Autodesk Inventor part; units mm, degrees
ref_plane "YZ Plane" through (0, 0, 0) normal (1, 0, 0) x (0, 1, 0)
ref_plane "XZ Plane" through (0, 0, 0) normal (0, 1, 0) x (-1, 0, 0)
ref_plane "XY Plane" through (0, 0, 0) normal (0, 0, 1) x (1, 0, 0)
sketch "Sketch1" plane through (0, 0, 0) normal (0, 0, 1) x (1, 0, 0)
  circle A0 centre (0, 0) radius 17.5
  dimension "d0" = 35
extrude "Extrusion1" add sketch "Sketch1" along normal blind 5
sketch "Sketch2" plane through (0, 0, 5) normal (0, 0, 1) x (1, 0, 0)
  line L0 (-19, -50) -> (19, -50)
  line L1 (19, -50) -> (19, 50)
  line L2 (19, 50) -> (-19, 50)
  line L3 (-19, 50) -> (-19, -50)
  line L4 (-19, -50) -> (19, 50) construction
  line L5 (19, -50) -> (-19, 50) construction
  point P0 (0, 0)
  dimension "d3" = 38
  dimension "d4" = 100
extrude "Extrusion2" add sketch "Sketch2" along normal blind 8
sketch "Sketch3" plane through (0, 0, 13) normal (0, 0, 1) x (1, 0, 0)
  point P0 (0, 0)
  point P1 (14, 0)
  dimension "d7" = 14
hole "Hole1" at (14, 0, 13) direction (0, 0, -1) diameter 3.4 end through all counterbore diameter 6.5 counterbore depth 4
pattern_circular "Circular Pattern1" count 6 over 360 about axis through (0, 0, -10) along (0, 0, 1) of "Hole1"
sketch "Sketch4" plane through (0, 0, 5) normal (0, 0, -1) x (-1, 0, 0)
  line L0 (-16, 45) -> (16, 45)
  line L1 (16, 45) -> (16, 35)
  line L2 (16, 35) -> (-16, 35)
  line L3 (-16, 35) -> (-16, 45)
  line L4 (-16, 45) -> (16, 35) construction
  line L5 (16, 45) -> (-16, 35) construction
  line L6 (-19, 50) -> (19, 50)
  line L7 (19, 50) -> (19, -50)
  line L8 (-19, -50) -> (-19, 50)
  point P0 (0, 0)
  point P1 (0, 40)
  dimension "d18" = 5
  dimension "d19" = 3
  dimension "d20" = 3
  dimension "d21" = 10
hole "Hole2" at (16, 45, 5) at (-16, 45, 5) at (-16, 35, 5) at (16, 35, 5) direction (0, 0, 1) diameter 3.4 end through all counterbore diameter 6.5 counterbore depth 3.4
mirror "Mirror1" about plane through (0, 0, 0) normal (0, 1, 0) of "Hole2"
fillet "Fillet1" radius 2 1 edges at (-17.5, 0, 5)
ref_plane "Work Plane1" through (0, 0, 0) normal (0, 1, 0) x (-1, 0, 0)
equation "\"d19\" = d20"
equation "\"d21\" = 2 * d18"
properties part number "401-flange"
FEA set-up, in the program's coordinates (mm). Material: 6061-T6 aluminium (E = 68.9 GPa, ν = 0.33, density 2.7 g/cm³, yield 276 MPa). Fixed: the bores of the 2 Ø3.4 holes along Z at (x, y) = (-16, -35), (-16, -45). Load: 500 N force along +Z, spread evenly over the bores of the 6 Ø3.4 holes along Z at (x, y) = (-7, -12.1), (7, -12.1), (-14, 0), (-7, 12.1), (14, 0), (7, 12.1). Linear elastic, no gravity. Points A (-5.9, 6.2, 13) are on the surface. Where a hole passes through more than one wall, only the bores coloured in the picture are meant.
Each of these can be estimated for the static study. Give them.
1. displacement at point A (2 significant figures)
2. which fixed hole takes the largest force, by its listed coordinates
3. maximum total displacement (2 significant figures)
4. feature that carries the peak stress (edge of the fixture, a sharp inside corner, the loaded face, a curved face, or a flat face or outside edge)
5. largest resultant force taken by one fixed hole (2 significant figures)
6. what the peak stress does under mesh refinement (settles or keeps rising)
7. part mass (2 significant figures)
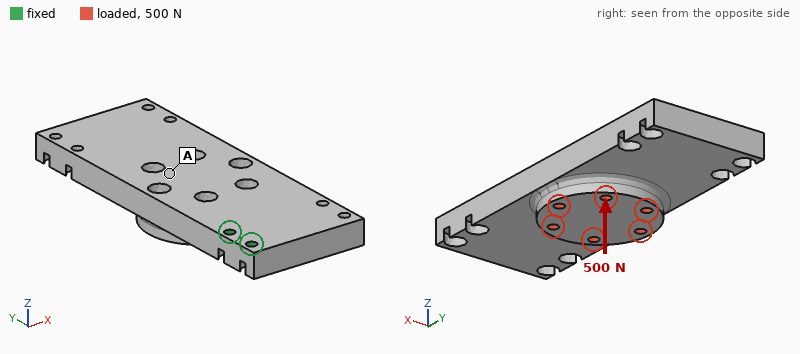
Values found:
0.23 mm
(-16, -35)
0.56 mm
edge of the fixture
1.5 kN
keeps rising
89 g
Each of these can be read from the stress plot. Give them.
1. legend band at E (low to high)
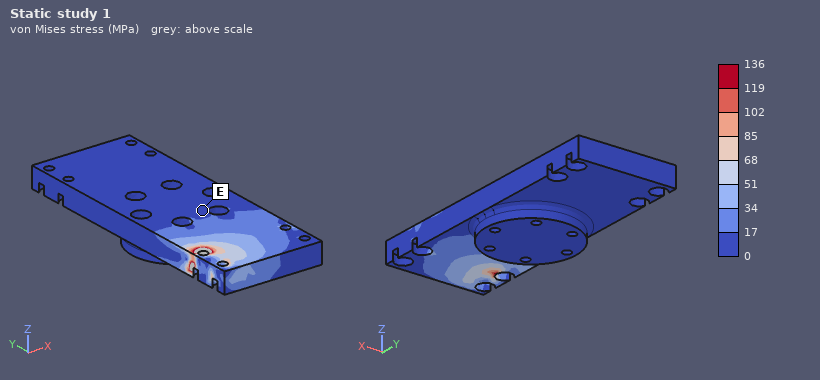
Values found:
0 to 17 MPa
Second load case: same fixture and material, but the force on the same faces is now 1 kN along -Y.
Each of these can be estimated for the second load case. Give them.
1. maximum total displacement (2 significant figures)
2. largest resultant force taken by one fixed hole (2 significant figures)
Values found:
0.15 mm
1.4 kN
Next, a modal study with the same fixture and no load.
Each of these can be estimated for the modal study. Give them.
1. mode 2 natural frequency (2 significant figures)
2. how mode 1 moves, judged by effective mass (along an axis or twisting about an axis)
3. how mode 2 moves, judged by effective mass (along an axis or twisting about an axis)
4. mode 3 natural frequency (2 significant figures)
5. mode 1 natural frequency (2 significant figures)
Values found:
1500 Hz
along Z
along X
2100 Hz
640 Hz
